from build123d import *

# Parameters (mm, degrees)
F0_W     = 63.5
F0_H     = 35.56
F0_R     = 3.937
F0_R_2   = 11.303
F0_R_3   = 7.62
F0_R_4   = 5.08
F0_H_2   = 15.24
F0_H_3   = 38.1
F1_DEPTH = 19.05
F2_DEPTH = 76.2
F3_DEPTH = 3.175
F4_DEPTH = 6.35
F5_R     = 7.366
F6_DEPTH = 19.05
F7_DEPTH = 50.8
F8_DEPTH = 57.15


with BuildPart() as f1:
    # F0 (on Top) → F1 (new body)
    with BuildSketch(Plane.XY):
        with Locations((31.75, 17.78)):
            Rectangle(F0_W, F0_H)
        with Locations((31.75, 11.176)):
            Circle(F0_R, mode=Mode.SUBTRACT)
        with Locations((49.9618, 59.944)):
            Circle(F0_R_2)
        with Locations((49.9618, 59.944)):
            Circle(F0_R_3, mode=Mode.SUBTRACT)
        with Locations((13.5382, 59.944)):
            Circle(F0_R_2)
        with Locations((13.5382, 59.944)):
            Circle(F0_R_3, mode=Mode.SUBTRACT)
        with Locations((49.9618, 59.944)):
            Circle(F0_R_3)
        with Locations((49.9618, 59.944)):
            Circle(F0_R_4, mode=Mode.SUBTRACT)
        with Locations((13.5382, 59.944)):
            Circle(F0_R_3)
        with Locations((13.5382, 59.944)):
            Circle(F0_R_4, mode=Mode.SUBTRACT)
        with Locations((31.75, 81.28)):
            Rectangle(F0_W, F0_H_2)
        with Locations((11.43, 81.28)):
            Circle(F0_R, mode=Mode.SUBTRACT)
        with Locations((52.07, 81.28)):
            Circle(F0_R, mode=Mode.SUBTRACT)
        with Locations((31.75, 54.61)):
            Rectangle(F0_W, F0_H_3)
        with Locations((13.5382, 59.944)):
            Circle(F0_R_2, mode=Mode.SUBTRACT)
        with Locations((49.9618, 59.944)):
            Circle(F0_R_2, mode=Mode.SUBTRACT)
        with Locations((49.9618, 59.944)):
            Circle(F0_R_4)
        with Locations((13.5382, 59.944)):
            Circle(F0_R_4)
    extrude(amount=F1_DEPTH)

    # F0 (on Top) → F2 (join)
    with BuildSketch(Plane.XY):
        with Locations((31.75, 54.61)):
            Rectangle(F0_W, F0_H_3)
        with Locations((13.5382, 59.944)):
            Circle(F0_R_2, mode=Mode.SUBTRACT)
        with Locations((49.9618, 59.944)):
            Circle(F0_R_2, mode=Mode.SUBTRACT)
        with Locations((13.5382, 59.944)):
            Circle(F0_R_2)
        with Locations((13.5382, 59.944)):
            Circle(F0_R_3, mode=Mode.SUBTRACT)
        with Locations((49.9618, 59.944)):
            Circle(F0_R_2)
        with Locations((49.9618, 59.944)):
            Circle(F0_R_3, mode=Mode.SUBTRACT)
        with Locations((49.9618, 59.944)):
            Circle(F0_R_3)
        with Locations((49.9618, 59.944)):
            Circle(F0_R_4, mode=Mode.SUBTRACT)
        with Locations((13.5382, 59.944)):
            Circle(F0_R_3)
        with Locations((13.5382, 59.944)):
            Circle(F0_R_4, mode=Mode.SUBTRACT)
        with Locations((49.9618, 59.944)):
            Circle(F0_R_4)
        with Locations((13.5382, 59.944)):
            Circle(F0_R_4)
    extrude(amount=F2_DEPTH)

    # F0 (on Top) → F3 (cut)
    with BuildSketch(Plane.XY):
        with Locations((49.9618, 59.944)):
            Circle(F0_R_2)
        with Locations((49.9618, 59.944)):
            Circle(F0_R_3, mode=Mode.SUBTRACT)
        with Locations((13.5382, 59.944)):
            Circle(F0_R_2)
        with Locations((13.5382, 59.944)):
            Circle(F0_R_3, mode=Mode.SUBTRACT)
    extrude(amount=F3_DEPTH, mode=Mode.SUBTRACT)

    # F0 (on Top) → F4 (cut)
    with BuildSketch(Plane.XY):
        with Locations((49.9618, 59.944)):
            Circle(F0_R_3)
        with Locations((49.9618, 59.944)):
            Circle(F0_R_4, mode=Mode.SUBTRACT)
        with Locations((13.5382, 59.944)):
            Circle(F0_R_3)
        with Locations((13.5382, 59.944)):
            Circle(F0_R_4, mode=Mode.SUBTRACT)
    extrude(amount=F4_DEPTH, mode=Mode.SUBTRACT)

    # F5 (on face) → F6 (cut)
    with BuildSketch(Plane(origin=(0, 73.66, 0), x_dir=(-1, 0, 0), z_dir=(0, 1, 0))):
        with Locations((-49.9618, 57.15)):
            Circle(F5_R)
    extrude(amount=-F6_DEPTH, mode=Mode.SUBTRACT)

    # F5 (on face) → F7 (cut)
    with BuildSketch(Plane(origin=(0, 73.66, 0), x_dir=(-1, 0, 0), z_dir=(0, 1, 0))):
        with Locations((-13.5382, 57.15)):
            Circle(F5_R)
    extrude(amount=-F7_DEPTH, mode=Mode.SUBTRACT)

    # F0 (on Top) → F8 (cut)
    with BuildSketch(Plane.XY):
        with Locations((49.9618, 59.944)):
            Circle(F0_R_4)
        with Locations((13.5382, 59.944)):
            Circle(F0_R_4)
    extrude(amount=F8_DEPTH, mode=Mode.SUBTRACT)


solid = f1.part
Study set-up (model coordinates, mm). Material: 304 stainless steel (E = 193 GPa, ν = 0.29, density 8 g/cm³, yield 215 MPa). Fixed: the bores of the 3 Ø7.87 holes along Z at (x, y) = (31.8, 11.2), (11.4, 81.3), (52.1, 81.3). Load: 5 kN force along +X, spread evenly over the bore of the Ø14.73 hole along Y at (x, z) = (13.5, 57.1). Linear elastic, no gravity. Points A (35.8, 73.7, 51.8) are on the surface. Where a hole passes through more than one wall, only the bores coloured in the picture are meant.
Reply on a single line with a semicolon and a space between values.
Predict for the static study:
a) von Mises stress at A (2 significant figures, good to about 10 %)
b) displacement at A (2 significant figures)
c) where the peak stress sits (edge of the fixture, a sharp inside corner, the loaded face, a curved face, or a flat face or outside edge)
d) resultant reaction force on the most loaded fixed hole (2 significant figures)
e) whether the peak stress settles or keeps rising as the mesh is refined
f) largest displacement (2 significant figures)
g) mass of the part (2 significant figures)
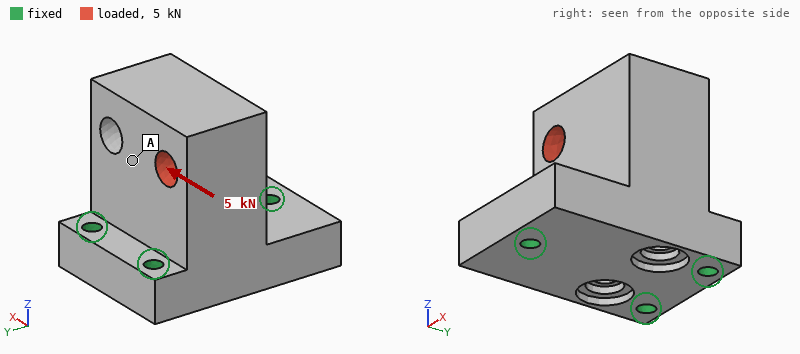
6.9 MPa; 7.8 µm; edge of the fixture; 4.9 kN; keeps rising; 13 µm; 1.8 kg
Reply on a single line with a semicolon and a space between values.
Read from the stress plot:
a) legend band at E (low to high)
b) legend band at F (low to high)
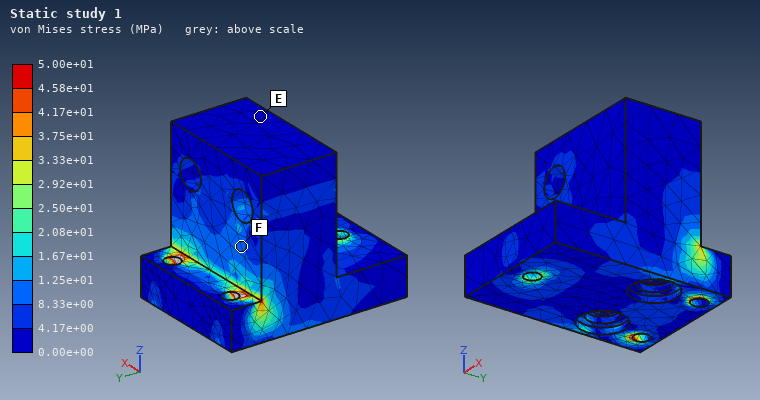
0.00e+00 to 4.17e+00 MPa; 8.33e+00 to 1.25e+01 MPa
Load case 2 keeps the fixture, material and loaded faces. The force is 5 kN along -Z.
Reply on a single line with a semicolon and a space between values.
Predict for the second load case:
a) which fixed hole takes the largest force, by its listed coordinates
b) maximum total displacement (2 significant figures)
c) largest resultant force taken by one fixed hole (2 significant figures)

(11.4, 81.3); 6.6 µm; 3.3 kN
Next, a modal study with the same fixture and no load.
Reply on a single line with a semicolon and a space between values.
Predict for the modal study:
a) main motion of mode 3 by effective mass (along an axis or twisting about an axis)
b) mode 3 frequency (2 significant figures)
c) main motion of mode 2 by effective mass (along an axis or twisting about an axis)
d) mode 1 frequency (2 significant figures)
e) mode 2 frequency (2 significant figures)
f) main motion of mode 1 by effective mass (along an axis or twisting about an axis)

along Z; 8600 Hz; along Y; 4100 Hz; 4300 Hz; along X
